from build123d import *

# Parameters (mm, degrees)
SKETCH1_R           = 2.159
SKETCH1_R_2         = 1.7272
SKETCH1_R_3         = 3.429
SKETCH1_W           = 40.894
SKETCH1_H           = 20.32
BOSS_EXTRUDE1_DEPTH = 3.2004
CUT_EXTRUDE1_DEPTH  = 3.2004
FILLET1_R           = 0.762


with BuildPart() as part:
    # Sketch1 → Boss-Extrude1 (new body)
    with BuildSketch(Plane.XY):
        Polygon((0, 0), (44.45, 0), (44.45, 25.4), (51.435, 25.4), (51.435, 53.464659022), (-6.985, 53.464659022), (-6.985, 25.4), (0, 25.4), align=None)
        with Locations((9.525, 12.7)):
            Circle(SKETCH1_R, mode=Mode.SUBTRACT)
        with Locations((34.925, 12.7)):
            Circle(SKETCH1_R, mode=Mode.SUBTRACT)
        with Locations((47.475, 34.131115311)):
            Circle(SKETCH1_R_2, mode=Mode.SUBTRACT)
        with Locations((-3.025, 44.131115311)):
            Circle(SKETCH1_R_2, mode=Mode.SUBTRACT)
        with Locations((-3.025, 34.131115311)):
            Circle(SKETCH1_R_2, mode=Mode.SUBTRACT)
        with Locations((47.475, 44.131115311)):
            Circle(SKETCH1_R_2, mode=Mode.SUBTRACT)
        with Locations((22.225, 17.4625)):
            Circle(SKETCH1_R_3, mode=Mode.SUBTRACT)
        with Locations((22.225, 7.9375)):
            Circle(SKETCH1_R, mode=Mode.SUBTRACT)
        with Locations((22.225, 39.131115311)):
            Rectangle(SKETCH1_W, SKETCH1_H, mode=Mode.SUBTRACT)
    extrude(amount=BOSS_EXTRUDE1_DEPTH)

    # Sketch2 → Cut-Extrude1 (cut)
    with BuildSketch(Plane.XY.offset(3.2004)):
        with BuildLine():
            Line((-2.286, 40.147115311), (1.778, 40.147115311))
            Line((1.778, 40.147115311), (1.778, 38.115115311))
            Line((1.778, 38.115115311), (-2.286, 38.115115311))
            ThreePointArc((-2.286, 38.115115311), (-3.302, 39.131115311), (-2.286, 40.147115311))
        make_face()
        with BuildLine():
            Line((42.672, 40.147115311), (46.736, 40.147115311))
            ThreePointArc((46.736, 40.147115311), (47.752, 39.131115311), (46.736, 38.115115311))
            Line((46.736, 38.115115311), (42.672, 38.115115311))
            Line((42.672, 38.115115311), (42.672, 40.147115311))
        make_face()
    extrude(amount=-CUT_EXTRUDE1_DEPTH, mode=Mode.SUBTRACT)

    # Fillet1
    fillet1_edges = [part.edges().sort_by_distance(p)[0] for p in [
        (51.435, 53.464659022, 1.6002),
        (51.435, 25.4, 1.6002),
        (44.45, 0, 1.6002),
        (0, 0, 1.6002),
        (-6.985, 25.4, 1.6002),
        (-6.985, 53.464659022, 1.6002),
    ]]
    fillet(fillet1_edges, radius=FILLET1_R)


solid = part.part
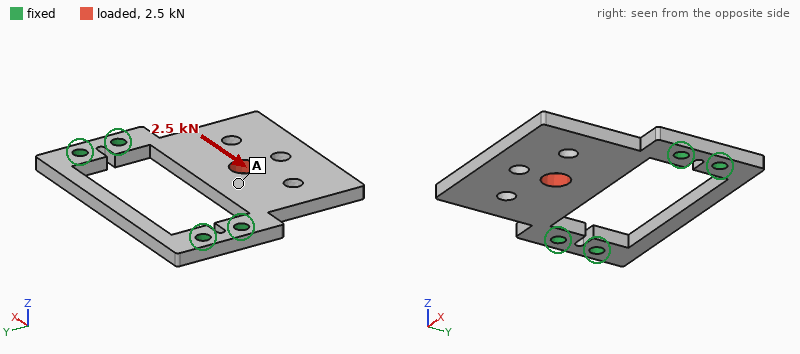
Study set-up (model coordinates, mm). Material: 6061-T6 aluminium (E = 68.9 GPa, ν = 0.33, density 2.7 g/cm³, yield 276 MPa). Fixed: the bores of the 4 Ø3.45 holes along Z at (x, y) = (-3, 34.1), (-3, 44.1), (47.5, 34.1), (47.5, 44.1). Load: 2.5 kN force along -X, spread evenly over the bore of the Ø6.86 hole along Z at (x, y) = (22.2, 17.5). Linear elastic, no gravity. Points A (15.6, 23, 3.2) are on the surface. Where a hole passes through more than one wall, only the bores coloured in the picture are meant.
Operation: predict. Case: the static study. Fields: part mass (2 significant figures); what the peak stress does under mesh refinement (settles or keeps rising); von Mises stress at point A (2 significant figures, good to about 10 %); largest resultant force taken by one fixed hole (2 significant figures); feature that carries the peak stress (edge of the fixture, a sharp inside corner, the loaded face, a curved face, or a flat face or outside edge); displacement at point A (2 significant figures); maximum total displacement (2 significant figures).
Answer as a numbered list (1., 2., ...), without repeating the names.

1. 16 g
2. keeps rising
3. 32 MPa
4. 1.4 kN
5. edge of the fixture
6. 33 µm
7. 39 µm
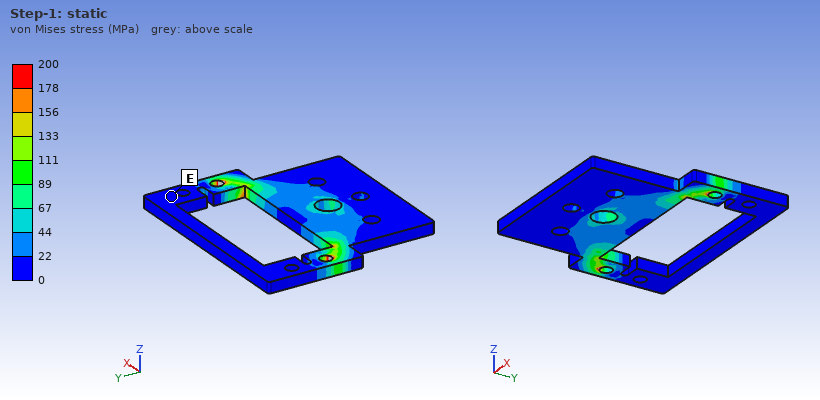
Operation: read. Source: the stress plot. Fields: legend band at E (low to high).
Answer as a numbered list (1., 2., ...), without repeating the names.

1. 0 to 22 MPa
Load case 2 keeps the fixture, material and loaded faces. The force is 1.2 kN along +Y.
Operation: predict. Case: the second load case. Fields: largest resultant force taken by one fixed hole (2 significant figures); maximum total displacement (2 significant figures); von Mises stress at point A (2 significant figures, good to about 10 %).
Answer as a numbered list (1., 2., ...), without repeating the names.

1. 690 N
2. 20 µm
3. 13 MPa
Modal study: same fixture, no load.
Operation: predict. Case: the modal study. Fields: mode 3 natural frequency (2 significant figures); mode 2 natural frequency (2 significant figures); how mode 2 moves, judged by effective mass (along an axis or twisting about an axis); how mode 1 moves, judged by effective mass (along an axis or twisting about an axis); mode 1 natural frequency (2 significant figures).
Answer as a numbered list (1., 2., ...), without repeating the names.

1. 6000 Hz
2. 4200 Hz
3. twisting about Y
4. along Z
5. 1300 Hz
